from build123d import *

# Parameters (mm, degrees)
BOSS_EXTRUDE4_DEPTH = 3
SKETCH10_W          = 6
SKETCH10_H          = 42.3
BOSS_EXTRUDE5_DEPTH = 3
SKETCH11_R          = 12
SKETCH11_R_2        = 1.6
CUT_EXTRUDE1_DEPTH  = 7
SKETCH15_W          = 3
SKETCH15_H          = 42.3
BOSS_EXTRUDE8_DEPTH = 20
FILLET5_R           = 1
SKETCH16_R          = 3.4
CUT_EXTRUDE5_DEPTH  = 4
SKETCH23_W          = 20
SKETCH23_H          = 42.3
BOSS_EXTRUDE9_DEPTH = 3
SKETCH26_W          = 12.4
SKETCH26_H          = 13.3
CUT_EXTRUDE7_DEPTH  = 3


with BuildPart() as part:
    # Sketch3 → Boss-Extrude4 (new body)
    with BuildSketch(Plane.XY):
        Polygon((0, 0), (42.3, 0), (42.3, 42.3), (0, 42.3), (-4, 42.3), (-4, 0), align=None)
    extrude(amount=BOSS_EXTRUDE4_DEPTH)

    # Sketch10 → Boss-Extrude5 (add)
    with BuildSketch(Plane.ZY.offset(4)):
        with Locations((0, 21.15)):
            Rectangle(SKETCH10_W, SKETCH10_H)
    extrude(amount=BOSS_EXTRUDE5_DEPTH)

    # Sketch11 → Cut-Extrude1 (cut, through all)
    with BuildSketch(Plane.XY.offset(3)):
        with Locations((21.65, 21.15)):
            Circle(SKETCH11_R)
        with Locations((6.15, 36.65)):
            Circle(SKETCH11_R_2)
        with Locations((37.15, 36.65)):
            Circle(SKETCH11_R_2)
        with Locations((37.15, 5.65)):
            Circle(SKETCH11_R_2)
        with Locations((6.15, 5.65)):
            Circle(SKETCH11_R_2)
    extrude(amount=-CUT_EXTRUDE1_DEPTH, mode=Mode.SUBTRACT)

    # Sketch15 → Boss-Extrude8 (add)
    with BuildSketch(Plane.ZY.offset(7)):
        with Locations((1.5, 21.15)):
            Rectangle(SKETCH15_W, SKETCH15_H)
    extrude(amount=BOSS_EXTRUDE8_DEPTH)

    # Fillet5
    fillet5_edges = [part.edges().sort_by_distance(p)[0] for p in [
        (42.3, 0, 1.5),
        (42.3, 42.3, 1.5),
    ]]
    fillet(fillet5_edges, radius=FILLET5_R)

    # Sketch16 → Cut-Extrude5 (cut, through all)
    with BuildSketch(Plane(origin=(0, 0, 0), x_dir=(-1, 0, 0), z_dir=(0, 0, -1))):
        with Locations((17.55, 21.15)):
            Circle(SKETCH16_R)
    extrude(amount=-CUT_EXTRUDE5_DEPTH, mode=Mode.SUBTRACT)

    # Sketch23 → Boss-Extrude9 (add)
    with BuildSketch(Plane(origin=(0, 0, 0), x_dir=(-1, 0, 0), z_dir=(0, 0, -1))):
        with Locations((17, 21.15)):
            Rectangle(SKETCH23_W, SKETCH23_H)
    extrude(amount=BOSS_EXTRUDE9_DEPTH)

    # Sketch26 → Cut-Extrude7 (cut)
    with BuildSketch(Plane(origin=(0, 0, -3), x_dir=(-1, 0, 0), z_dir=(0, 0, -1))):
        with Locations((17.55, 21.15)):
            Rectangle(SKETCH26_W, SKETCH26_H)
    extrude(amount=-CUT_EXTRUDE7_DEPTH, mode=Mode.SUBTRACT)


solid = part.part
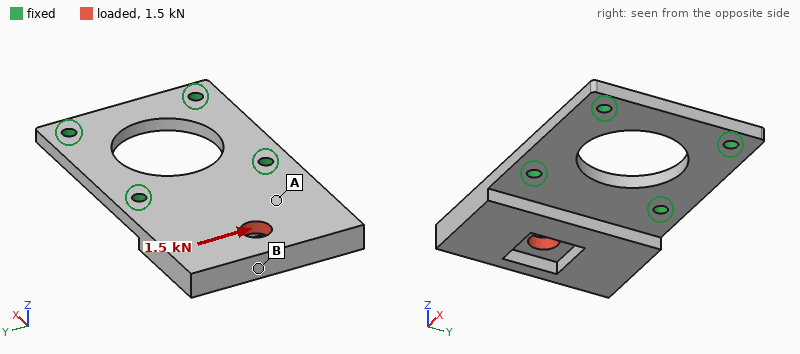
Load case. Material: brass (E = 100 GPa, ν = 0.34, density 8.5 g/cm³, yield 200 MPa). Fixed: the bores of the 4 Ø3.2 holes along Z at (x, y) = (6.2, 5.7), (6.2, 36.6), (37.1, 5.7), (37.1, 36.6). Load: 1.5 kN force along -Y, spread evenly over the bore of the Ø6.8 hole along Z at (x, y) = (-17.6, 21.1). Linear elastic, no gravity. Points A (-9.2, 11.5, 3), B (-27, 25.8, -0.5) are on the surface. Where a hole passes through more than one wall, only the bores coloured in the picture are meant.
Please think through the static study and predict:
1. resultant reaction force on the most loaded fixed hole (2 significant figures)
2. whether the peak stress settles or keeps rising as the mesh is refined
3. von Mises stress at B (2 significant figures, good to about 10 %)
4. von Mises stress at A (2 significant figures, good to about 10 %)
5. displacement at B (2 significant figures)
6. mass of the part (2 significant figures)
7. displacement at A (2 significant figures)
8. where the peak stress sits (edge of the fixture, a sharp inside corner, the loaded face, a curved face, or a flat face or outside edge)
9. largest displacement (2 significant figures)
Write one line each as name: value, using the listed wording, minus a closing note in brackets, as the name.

resultant reaction force on the most loaded fixed hole: 1.3 kN
whether the peak stress settles or keeps rising as the mesh is refined: keeps rising
von Mises stress at B: 10 MPa
von Mises stress at A: 25 MPa
displacement at B: 15 µm
mass of the part: 82 g
displacement at A: 8.9 µm
where the peak stress sits: edge of the fixture
largest displacement: 22 µm
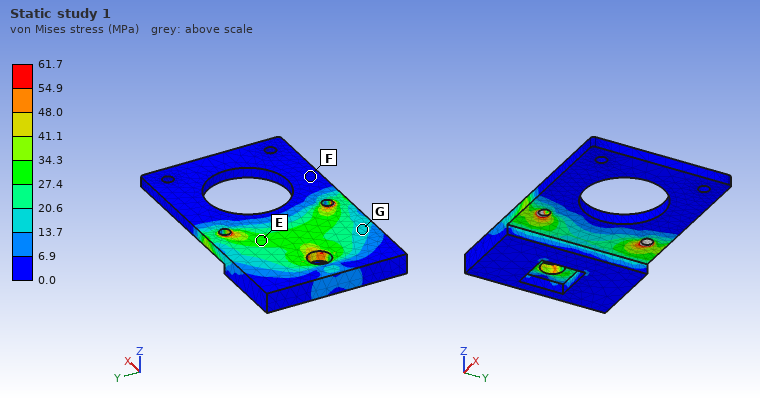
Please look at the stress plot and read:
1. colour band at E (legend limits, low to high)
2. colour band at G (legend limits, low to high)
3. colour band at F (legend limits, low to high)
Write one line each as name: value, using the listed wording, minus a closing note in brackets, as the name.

colour band at E: 27.4 to 34.3 MPa
colour band at G: 13.7 to 20.6 MPa
colour band at F: 0.0 to 6.9 MPa
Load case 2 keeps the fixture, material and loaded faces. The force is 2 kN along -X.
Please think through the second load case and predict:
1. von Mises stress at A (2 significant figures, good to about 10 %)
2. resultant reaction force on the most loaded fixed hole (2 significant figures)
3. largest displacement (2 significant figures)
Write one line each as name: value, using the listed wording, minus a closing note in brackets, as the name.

von Mises stress at A: 22 MPa
resultant reaction force on the most loaded fixed hole: 990 N
largest displacement: 11 µm
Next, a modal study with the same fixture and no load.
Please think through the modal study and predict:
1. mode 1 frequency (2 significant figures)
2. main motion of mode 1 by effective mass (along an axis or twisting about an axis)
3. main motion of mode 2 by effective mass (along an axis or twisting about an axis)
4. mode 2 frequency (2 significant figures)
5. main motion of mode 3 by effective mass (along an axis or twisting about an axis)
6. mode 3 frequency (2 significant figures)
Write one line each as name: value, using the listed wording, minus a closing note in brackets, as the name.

mode 1 frequency: 1100 Hz
main motion of mode 1 by effective mass: along Z
main motion of mode 2 by effective mass: twisting about X
mode 2 frequency: 3500 Hz
main motion of mode 3 by effective mass: along Y
mode 3 frequency: 8500 Hz
